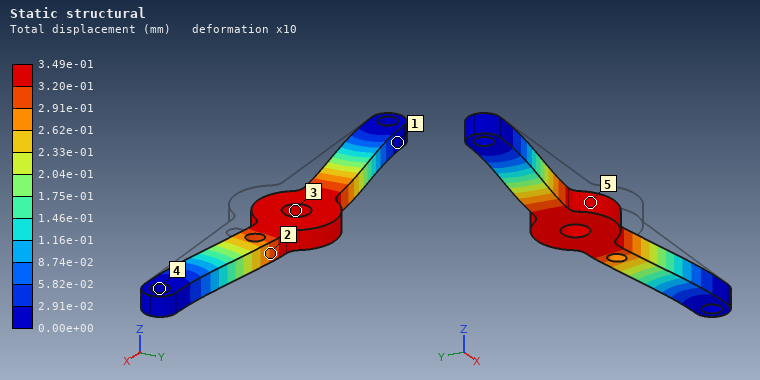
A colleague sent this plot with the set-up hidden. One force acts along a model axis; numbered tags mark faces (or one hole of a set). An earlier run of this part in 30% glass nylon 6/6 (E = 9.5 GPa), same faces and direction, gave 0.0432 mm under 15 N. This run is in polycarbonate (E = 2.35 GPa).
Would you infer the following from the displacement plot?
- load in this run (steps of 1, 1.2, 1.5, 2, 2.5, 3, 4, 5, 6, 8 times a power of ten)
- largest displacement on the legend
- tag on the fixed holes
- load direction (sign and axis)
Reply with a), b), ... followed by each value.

a) 30 N
b) 3.49e-01 mm
c) 4
d) +Y
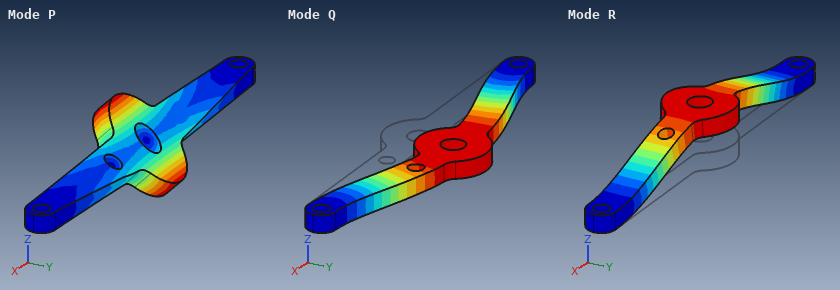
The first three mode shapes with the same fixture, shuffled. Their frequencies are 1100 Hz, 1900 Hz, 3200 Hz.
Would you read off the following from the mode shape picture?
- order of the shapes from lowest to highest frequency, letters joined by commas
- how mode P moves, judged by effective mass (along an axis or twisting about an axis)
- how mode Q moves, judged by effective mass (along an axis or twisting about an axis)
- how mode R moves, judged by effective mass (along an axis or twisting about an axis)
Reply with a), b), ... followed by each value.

a) R, Q, P
b) twisting about X
c) along Y
d) along Z
